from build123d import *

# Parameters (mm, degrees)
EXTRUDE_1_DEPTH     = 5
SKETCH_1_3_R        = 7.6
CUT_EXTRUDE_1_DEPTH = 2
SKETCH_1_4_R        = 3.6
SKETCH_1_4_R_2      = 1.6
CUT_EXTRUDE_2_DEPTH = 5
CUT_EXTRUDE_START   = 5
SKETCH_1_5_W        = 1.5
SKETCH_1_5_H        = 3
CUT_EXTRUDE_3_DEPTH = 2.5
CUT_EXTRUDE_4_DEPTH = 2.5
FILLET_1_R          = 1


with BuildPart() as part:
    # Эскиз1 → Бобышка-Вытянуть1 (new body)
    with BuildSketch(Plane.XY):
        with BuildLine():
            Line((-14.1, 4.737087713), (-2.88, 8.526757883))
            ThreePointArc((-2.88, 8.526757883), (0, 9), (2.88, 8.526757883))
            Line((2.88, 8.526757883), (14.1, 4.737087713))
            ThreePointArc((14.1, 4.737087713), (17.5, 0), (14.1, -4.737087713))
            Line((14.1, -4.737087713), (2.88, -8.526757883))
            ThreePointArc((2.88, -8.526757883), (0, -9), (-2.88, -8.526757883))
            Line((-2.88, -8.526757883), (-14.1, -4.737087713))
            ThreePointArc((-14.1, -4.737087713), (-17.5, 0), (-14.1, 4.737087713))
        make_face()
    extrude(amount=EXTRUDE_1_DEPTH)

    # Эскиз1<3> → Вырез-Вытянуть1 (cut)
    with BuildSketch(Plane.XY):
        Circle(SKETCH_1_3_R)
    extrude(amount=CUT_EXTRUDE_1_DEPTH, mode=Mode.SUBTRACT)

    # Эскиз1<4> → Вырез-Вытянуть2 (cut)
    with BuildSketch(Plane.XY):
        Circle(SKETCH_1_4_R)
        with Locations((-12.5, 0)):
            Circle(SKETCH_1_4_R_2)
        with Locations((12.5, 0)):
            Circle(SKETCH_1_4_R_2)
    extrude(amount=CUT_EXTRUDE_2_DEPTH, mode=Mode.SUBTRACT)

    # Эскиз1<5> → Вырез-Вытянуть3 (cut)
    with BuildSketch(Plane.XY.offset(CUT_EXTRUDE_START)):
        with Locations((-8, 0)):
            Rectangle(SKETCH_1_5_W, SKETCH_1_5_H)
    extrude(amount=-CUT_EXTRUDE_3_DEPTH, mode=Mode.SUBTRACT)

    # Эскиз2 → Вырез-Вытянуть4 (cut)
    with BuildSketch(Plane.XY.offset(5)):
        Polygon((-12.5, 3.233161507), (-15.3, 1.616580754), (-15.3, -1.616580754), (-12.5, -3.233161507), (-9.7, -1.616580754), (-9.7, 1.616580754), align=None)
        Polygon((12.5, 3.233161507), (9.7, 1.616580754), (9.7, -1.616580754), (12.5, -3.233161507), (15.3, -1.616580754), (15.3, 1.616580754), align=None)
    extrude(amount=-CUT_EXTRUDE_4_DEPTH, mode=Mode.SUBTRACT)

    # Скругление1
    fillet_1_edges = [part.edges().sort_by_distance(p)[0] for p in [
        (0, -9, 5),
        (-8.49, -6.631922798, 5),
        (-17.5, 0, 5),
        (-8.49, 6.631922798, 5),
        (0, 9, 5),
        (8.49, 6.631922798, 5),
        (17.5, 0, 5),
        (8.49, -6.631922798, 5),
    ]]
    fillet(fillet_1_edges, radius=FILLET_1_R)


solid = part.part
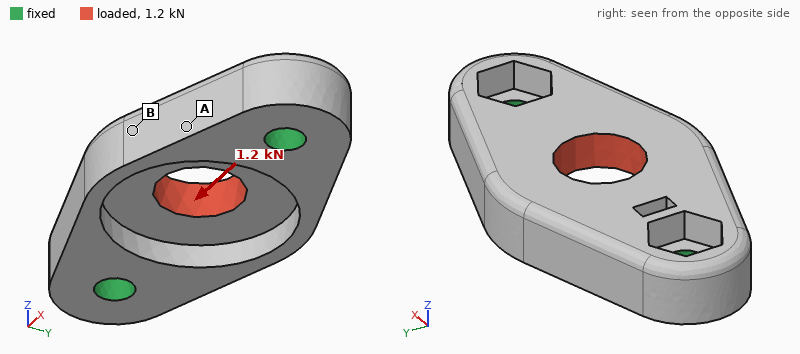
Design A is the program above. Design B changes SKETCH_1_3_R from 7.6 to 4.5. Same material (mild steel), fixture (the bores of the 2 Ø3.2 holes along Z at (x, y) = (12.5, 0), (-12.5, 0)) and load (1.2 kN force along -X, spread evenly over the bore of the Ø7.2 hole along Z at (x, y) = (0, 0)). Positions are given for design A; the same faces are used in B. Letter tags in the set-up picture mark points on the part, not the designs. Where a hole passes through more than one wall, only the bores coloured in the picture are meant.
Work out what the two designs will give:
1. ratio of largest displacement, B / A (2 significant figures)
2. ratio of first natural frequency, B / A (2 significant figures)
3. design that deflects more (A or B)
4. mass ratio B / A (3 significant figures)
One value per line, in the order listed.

0.77
0.98
A
1.15
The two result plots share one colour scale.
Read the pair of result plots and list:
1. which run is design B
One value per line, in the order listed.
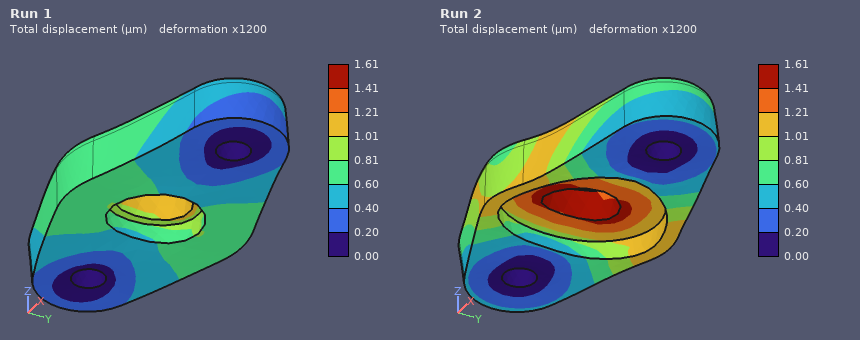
Run 1
